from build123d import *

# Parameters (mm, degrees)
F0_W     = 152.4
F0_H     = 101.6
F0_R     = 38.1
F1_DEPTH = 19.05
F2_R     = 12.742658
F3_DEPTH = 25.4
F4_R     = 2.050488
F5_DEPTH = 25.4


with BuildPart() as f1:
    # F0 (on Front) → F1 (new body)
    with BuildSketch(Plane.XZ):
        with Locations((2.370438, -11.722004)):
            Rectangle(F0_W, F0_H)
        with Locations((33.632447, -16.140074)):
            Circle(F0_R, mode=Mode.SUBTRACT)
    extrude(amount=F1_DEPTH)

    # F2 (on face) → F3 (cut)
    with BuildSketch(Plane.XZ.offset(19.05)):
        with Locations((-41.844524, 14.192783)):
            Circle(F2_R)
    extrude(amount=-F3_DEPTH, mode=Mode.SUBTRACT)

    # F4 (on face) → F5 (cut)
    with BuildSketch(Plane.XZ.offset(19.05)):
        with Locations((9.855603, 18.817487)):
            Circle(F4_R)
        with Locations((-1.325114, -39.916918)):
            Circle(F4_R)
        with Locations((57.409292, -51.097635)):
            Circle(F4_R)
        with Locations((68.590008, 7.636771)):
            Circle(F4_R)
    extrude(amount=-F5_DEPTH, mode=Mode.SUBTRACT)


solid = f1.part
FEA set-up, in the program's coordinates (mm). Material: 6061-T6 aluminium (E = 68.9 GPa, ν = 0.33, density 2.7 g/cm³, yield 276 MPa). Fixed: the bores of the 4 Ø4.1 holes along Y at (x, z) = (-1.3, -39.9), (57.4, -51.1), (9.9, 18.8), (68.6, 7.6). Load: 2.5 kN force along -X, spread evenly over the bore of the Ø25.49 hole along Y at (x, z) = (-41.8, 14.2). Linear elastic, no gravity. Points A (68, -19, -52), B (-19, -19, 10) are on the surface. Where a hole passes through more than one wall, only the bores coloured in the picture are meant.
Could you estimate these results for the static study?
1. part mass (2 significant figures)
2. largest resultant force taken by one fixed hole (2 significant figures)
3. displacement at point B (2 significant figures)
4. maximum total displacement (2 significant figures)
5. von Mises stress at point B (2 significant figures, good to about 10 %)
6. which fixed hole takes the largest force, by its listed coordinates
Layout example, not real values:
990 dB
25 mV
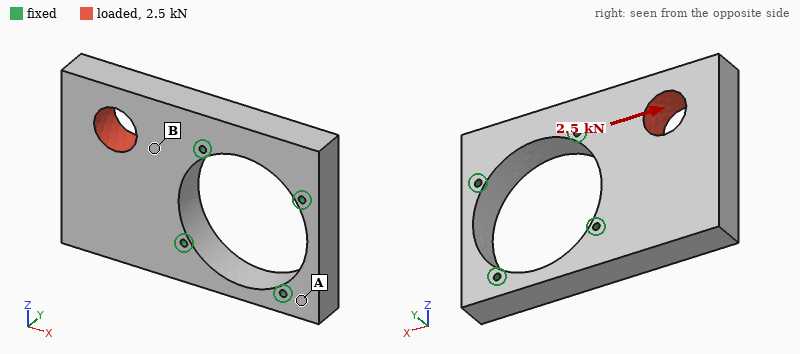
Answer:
530 g
2.0 kN
1.9 µm
4.8 µm
3.1 MPa
(9.9, 18.8)
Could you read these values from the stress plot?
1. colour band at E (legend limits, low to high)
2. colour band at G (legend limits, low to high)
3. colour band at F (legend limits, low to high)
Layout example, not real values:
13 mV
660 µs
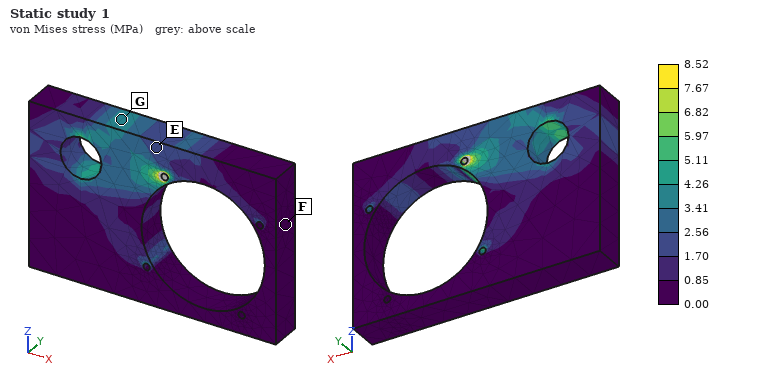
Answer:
1.70 to 2.56 MPa
3.41 to 4.26 MPa
0.00 to 0.85 MPa
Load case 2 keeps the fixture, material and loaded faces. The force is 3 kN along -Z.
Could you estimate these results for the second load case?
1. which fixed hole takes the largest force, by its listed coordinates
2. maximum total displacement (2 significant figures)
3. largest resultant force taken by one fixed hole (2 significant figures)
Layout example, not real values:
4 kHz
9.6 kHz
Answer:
(-1.3, -39.9)
11 µm
2.4 kN
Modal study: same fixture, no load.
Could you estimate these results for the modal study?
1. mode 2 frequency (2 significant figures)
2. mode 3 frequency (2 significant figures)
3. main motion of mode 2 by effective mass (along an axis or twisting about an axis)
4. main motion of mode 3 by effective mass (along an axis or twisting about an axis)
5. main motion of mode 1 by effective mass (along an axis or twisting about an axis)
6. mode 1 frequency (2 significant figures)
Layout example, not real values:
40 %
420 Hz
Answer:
3900 Hz
5500 Hz
twisting about X
along Z
along Y
1800 Hz
